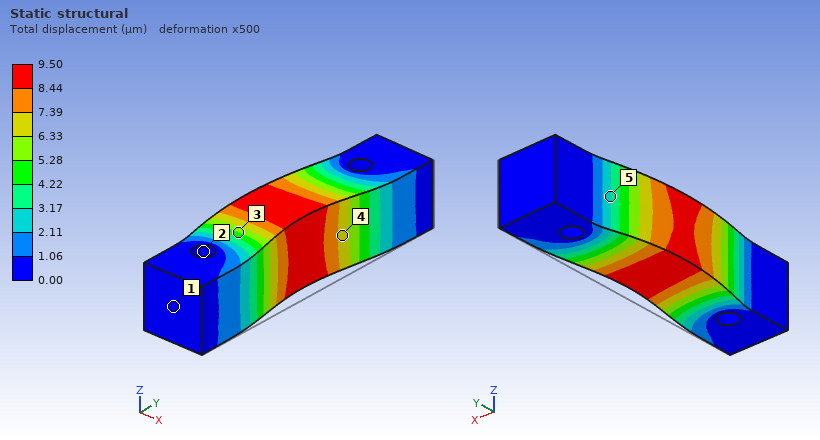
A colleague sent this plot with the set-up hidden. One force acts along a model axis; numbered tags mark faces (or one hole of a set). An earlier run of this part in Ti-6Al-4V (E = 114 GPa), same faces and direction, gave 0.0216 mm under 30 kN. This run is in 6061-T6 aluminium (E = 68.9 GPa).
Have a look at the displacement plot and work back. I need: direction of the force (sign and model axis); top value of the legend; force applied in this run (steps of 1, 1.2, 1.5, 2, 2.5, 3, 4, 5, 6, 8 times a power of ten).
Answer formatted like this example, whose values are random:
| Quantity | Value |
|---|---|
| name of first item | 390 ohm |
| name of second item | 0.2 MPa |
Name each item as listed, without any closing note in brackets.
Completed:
| Quantity | Value |
|---|---|
| direction of the force | -X |
| top value of the legend | 9.50 µm |
| force applied in this run | 8 kN |
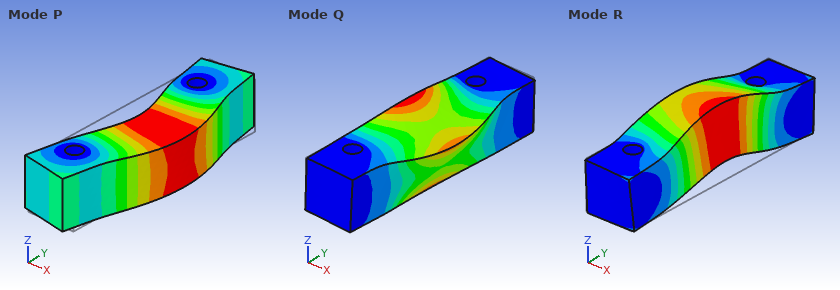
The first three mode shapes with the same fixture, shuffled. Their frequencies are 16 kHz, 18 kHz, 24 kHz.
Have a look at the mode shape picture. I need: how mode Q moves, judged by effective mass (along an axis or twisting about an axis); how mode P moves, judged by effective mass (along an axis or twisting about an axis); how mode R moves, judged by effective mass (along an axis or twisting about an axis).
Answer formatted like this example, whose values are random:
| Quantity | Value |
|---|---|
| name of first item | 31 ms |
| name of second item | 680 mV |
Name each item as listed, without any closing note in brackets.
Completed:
| Quantity | Value |
|---|---|
| how mode Q moves, judged by effective mass | twisting about Y |
| how mode P moves, judged by effective mass | along X |
| how mode R moves, judged by effective mass | along Z |
